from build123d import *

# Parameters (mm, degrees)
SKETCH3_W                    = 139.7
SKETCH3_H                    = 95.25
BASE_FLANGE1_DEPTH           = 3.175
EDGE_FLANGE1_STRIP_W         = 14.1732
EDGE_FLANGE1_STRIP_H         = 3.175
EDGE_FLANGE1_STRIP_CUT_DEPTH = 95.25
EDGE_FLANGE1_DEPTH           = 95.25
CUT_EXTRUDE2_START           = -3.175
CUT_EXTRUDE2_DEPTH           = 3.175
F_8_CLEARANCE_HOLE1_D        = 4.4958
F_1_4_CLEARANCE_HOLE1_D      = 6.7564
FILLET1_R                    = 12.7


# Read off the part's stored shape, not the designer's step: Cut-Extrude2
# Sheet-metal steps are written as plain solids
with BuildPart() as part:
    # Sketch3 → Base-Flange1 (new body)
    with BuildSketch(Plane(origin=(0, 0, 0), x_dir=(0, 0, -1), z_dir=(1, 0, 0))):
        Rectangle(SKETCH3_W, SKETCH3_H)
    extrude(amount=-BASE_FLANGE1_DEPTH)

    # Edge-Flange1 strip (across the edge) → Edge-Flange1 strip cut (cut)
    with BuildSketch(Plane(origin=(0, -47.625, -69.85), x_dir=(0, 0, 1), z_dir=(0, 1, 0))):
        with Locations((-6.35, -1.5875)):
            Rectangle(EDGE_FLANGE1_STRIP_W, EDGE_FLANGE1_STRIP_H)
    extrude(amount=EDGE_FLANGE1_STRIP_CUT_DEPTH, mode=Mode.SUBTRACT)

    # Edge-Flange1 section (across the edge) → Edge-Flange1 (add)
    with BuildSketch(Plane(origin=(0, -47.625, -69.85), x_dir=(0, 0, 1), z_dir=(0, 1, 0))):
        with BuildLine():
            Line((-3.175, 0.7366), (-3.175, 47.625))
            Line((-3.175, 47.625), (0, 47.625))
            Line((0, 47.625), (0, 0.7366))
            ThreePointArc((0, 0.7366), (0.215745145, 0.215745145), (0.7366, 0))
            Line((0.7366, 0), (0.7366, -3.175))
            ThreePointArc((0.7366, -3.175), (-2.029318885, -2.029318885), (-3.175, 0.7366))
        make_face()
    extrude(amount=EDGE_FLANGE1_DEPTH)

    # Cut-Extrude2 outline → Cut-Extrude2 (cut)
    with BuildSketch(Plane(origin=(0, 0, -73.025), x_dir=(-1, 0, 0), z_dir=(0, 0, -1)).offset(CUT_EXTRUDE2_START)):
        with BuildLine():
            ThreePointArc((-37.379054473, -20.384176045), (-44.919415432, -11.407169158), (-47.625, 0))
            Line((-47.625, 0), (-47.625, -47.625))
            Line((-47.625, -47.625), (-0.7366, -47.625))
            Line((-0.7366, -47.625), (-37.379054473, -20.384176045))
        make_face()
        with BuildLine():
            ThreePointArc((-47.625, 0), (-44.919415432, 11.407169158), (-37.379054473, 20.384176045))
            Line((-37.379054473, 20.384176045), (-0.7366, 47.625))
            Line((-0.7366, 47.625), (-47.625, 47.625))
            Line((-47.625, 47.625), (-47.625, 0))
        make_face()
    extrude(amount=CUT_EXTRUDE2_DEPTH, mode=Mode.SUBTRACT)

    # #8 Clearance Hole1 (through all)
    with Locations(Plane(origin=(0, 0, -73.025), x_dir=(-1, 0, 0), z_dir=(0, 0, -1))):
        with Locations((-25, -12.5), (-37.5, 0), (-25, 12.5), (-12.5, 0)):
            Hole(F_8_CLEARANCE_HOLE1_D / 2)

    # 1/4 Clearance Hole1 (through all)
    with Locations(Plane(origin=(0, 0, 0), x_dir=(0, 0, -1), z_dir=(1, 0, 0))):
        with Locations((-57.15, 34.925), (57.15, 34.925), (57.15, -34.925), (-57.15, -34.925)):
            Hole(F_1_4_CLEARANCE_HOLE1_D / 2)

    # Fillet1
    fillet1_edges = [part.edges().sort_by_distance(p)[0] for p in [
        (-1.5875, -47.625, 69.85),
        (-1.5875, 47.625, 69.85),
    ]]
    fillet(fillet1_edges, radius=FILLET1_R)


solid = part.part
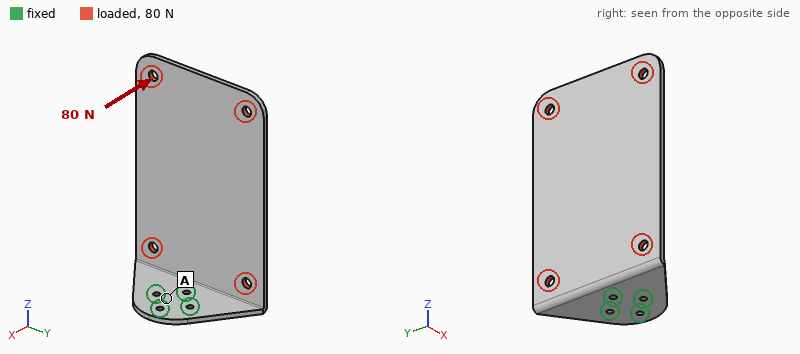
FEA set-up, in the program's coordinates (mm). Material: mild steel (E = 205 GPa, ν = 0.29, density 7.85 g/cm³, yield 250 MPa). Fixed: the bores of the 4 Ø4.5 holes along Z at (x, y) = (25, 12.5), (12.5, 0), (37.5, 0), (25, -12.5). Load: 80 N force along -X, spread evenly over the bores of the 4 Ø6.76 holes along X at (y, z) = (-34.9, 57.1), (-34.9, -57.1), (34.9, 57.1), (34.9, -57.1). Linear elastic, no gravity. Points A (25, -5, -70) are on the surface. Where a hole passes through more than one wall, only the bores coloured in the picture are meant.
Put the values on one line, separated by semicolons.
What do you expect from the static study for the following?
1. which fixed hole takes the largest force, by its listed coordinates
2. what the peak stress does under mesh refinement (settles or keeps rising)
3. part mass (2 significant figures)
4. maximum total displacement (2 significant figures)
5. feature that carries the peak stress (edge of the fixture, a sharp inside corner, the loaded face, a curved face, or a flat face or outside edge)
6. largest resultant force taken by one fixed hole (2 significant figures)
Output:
(12.5, 0); keeps rising; 400 g; 0.91 mm; edge of the fixture; 270 N
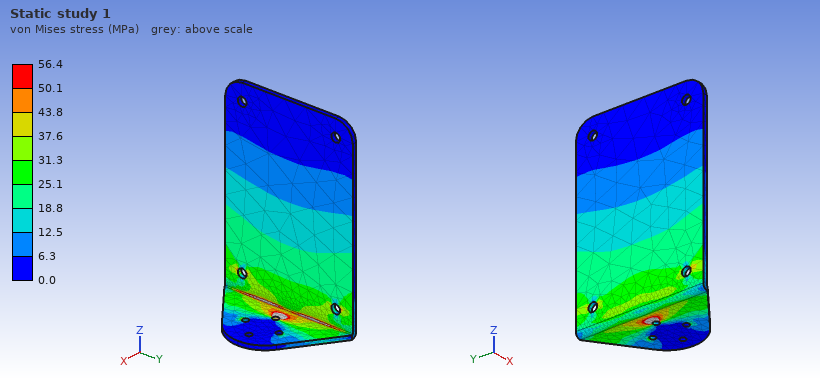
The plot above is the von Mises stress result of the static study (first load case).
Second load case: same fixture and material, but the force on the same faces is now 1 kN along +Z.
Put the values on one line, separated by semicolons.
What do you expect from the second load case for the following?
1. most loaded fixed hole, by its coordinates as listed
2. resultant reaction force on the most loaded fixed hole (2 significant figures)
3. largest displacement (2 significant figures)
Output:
(12.5, 0); 1.3 kN; 0.48 mm
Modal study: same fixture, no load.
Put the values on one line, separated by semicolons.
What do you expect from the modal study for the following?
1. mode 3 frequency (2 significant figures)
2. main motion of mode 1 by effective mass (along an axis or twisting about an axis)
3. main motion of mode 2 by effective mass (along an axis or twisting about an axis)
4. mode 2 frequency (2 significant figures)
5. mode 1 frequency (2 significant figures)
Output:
430 Hz; along X; along Y; 230 Hz; 110 Hz
